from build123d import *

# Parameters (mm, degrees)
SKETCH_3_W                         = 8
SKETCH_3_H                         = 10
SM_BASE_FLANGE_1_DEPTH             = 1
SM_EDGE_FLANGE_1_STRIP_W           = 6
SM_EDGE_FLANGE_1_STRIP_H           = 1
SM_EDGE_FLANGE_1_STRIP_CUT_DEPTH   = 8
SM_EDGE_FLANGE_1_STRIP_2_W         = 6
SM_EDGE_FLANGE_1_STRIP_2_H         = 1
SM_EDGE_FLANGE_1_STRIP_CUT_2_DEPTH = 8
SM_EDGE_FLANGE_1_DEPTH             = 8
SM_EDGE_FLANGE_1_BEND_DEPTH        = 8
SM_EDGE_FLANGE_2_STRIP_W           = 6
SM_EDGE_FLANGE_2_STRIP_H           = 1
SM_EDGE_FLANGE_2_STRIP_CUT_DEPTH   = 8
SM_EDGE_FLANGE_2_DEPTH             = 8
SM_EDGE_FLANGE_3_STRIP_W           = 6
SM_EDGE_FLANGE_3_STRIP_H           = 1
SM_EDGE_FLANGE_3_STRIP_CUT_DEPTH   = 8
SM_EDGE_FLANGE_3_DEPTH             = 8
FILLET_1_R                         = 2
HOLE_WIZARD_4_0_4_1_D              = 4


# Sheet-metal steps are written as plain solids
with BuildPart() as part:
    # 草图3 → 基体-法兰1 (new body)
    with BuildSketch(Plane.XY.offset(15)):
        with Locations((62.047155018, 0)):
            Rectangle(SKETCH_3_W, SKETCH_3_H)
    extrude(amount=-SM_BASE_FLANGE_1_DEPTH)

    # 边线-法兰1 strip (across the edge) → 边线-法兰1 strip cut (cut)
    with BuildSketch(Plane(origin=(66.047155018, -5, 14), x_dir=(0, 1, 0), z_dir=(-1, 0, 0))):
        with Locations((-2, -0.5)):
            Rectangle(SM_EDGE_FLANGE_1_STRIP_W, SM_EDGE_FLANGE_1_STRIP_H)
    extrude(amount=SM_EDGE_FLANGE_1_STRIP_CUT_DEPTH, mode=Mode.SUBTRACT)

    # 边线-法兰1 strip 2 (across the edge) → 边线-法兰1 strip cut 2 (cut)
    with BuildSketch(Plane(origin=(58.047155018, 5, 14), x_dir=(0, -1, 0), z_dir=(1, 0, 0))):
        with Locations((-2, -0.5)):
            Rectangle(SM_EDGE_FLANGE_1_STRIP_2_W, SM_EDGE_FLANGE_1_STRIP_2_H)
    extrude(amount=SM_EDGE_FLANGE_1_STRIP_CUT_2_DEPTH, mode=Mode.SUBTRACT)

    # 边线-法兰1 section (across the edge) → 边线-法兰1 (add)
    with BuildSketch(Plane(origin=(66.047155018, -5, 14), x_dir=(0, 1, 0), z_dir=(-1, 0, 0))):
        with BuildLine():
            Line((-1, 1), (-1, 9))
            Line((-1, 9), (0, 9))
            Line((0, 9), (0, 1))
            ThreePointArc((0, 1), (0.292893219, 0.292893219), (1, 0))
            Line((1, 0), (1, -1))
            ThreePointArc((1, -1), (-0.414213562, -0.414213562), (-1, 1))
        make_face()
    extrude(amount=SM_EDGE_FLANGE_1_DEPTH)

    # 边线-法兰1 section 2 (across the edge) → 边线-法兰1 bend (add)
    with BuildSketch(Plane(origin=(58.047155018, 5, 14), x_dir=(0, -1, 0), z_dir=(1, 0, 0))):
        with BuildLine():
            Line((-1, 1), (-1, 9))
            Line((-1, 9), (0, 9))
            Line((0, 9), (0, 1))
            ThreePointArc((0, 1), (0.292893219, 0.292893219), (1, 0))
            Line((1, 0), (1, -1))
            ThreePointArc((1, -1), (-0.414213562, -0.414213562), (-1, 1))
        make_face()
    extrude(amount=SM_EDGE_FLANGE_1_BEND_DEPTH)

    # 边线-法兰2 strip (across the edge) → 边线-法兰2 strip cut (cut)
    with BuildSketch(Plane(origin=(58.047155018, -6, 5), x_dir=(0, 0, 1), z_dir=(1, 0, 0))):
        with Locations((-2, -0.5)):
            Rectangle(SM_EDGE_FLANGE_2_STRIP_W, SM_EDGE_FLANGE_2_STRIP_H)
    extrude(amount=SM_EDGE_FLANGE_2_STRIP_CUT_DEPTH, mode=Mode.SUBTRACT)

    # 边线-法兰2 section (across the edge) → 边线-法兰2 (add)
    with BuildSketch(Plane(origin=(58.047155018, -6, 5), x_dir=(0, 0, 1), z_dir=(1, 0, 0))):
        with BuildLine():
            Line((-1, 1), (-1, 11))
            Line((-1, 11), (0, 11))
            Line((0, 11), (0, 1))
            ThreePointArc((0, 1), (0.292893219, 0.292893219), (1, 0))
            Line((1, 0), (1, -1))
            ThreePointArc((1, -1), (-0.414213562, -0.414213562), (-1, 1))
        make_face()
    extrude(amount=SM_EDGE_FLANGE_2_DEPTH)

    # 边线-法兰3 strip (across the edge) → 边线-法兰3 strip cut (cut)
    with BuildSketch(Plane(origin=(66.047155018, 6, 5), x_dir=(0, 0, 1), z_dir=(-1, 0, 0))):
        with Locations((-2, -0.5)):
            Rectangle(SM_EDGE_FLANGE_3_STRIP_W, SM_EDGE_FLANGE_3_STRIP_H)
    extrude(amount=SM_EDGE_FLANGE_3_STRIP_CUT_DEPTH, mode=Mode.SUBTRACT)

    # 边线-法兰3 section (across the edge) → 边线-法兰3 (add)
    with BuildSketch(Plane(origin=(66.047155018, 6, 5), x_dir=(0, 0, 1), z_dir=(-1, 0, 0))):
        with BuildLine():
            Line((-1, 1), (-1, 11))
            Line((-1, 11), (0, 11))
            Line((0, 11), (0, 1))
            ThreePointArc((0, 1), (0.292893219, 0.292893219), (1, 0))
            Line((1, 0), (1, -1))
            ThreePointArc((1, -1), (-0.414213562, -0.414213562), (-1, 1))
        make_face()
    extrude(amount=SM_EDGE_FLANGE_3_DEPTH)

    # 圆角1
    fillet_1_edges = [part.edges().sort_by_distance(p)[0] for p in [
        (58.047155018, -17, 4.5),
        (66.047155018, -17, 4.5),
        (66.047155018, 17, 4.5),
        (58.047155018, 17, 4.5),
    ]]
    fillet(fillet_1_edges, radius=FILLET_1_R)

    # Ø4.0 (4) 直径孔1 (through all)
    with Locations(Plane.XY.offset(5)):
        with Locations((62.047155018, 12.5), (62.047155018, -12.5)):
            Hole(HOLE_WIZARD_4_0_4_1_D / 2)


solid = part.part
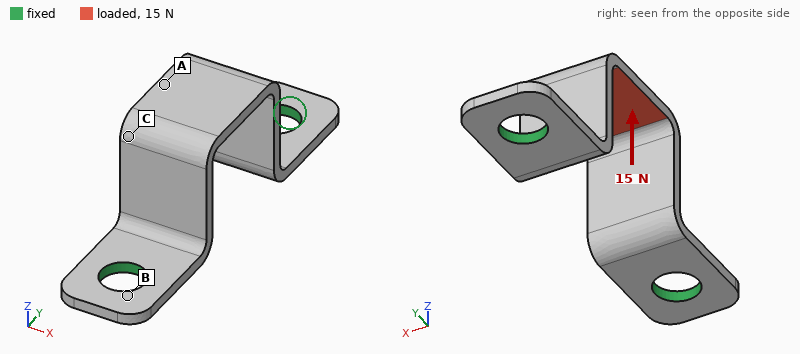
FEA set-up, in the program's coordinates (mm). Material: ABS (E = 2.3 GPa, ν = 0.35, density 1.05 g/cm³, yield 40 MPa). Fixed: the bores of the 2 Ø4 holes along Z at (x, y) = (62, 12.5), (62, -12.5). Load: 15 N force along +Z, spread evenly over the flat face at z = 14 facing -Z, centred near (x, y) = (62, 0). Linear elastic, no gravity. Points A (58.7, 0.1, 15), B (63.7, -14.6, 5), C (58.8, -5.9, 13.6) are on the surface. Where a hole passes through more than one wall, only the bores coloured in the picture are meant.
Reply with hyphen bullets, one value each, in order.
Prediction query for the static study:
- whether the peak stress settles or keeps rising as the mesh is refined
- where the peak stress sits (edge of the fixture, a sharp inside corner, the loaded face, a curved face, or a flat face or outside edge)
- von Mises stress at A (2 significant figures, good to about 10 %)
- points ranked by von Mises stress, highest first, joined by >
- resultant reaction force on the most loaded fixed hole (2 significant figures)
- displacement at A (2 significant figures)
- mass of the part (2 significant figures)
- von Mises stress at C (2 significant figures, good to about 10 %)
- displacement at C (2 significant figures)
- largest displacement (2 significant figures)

- keeps rising
- edge of the fixture
- 8.7 MPa
- A > C > B
- 8.2 N
- 0.17 mm
- 0.40 g
- 5.8 MPa
- 0.100 mm
- 0.17 mm
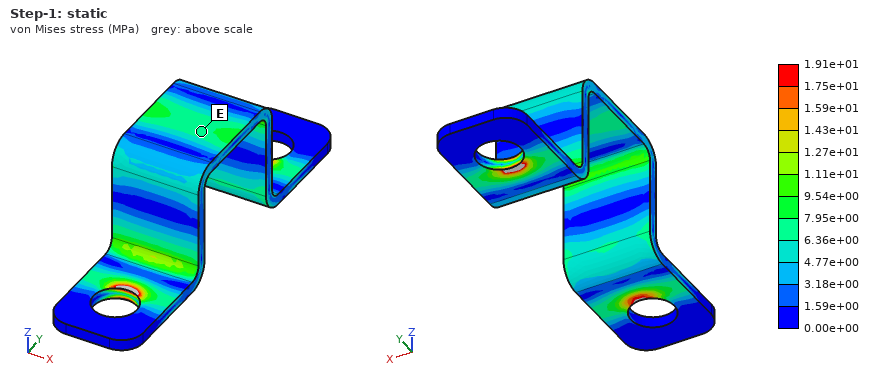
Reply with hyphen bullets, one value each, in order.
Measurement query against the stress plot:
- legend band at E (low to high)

- 6.36e+00 to 7.95e+00 MPa
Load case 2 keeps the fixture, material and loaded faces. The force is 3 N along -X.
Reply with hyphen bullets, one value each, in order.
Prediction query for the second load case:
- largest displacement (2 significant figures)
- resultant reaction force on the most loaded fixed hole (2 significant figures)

- 0.26 mm
- 1.5 N
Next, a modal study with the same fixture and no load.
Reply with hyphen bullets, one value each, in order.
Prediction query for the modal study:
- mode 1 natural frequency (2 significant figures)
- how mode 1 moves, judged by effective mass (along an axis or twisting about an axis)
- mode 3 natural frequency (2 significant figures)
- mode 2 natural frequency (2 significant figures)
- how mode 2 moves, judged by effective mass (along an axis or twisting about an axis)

- 1400 Hz
- along X
- 3000 Hz
- 2000 Hz
- along Y
